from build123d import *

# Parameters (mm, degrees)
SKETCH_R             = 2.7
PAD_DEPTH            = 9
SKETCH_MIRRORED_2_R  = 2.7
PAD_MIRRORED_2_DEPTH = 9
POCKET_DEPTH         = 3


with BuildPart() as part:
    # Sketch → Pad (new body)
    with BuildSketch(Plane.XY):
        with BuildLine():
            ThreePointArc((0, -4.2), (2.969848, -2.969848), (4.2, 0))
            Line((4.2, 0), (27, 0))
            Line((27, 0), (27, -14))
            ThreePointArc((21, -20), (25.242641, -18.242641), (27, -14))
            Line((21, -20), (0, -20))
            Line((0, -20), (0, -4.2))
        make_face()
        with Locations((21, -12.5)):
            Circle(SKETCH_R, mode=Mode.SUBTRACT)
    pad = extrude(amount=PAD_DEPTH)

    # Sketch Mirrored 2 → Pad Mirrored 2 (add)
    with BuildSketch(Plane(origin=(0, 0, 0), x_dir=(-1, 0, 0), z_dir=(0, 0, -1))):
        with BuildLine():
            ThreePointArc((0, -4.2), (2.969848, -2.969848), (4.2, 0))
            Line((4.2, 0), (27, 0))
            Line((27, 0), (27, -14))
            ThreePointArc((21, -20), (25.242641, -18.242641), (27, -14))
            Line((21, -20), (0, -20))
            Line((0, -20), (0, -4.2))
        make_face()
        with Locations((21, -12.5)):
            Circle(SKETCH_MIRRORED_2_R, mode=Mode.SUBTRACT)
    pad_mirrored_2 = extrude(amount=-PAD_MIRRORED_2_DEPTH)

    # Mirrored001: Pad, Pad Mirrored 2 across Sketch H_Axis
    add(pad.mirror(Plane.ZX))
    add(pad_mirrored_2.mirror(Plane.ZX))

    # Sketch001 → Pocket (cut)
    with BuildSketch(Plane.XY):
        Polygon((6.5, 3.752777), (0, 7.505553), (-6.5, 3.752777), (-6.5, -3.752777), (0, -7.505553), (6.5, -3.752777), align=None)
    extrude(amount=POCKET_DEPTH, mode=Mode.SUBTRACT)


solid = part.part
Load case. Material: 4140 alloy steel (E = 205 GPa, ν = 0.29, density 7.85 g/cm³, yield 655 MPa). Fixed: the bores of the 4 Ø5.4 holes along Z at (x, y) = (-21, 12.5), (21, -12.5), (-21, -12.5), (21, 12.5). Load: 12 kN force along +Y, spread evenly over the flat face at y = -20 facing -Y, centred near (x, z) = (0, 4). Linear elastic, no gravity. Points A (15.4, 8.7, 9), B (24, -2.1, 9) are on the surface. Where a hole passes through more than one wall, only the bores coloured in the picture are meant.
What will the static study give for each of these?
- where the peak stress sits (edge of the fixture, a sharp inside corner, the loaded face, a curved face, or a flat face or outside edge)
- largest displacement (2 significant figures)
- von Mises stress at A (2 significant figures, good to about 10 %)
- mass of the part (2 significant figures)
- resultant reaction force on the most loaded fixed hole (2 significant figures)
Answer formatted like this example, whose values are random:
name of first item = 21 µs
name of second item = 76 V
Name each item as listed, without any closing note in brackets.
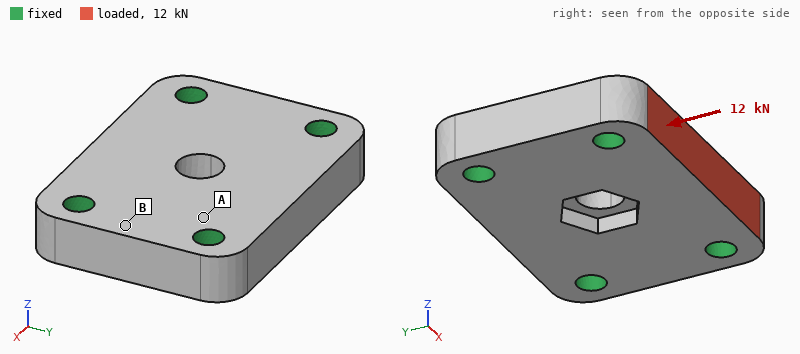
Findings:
where the peak stress sits = edge of the fixture
largest displacement = 5.5 µm
von Mises stress at A = 26 MPa
mass of the part = 140 g
resultant reaction force on the most loaded fixed hole = 4.1 kN
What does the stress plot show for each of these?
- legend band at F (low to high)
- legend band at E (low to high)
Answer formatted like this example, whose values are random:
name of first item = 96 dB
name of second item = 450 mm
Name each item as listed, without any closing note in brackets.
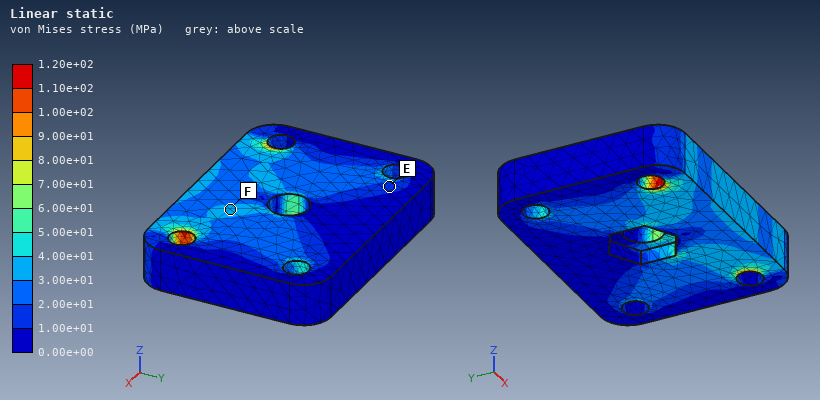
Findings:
legend band at F = 3.00e+01 to 4.00e+01 MPa
legend band at E = 1.00e+01 to 2.00e+01 MPa
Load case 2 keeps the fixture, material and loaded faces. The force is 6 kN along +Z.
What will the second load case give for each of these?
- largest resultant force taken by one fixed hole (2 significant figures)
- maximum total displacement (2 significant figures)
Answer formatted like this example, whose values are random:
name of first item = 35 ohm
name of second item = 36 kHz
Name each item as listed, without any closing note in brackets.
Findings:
largest resultant force taken by one fixed hole = 3.3 kN
maximum total displacement = 17 µm
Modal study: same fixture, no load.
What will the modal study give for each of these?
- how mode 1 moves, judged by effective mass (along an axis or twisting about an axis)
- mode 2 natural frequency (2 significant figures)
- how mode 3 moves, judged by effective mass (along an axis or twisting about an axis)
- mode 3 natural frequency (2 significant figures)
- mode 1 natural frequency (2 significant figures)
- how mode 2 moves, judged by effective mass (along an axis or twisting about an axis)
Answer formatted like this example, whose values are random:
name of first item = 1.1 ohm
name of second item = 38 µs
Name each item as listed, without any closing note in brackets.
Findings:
how mode 1 moves, judged by effective mass = along Z
mode 2 natural frequency = 26 kHz
how mode 3 moves, judged by effective mass = along Y
mode 3 natural frequency = 35 kHz
mode 1 natural frequency = 21 kHz
how mode 2 moves, judged by effective mass = twisting about X
